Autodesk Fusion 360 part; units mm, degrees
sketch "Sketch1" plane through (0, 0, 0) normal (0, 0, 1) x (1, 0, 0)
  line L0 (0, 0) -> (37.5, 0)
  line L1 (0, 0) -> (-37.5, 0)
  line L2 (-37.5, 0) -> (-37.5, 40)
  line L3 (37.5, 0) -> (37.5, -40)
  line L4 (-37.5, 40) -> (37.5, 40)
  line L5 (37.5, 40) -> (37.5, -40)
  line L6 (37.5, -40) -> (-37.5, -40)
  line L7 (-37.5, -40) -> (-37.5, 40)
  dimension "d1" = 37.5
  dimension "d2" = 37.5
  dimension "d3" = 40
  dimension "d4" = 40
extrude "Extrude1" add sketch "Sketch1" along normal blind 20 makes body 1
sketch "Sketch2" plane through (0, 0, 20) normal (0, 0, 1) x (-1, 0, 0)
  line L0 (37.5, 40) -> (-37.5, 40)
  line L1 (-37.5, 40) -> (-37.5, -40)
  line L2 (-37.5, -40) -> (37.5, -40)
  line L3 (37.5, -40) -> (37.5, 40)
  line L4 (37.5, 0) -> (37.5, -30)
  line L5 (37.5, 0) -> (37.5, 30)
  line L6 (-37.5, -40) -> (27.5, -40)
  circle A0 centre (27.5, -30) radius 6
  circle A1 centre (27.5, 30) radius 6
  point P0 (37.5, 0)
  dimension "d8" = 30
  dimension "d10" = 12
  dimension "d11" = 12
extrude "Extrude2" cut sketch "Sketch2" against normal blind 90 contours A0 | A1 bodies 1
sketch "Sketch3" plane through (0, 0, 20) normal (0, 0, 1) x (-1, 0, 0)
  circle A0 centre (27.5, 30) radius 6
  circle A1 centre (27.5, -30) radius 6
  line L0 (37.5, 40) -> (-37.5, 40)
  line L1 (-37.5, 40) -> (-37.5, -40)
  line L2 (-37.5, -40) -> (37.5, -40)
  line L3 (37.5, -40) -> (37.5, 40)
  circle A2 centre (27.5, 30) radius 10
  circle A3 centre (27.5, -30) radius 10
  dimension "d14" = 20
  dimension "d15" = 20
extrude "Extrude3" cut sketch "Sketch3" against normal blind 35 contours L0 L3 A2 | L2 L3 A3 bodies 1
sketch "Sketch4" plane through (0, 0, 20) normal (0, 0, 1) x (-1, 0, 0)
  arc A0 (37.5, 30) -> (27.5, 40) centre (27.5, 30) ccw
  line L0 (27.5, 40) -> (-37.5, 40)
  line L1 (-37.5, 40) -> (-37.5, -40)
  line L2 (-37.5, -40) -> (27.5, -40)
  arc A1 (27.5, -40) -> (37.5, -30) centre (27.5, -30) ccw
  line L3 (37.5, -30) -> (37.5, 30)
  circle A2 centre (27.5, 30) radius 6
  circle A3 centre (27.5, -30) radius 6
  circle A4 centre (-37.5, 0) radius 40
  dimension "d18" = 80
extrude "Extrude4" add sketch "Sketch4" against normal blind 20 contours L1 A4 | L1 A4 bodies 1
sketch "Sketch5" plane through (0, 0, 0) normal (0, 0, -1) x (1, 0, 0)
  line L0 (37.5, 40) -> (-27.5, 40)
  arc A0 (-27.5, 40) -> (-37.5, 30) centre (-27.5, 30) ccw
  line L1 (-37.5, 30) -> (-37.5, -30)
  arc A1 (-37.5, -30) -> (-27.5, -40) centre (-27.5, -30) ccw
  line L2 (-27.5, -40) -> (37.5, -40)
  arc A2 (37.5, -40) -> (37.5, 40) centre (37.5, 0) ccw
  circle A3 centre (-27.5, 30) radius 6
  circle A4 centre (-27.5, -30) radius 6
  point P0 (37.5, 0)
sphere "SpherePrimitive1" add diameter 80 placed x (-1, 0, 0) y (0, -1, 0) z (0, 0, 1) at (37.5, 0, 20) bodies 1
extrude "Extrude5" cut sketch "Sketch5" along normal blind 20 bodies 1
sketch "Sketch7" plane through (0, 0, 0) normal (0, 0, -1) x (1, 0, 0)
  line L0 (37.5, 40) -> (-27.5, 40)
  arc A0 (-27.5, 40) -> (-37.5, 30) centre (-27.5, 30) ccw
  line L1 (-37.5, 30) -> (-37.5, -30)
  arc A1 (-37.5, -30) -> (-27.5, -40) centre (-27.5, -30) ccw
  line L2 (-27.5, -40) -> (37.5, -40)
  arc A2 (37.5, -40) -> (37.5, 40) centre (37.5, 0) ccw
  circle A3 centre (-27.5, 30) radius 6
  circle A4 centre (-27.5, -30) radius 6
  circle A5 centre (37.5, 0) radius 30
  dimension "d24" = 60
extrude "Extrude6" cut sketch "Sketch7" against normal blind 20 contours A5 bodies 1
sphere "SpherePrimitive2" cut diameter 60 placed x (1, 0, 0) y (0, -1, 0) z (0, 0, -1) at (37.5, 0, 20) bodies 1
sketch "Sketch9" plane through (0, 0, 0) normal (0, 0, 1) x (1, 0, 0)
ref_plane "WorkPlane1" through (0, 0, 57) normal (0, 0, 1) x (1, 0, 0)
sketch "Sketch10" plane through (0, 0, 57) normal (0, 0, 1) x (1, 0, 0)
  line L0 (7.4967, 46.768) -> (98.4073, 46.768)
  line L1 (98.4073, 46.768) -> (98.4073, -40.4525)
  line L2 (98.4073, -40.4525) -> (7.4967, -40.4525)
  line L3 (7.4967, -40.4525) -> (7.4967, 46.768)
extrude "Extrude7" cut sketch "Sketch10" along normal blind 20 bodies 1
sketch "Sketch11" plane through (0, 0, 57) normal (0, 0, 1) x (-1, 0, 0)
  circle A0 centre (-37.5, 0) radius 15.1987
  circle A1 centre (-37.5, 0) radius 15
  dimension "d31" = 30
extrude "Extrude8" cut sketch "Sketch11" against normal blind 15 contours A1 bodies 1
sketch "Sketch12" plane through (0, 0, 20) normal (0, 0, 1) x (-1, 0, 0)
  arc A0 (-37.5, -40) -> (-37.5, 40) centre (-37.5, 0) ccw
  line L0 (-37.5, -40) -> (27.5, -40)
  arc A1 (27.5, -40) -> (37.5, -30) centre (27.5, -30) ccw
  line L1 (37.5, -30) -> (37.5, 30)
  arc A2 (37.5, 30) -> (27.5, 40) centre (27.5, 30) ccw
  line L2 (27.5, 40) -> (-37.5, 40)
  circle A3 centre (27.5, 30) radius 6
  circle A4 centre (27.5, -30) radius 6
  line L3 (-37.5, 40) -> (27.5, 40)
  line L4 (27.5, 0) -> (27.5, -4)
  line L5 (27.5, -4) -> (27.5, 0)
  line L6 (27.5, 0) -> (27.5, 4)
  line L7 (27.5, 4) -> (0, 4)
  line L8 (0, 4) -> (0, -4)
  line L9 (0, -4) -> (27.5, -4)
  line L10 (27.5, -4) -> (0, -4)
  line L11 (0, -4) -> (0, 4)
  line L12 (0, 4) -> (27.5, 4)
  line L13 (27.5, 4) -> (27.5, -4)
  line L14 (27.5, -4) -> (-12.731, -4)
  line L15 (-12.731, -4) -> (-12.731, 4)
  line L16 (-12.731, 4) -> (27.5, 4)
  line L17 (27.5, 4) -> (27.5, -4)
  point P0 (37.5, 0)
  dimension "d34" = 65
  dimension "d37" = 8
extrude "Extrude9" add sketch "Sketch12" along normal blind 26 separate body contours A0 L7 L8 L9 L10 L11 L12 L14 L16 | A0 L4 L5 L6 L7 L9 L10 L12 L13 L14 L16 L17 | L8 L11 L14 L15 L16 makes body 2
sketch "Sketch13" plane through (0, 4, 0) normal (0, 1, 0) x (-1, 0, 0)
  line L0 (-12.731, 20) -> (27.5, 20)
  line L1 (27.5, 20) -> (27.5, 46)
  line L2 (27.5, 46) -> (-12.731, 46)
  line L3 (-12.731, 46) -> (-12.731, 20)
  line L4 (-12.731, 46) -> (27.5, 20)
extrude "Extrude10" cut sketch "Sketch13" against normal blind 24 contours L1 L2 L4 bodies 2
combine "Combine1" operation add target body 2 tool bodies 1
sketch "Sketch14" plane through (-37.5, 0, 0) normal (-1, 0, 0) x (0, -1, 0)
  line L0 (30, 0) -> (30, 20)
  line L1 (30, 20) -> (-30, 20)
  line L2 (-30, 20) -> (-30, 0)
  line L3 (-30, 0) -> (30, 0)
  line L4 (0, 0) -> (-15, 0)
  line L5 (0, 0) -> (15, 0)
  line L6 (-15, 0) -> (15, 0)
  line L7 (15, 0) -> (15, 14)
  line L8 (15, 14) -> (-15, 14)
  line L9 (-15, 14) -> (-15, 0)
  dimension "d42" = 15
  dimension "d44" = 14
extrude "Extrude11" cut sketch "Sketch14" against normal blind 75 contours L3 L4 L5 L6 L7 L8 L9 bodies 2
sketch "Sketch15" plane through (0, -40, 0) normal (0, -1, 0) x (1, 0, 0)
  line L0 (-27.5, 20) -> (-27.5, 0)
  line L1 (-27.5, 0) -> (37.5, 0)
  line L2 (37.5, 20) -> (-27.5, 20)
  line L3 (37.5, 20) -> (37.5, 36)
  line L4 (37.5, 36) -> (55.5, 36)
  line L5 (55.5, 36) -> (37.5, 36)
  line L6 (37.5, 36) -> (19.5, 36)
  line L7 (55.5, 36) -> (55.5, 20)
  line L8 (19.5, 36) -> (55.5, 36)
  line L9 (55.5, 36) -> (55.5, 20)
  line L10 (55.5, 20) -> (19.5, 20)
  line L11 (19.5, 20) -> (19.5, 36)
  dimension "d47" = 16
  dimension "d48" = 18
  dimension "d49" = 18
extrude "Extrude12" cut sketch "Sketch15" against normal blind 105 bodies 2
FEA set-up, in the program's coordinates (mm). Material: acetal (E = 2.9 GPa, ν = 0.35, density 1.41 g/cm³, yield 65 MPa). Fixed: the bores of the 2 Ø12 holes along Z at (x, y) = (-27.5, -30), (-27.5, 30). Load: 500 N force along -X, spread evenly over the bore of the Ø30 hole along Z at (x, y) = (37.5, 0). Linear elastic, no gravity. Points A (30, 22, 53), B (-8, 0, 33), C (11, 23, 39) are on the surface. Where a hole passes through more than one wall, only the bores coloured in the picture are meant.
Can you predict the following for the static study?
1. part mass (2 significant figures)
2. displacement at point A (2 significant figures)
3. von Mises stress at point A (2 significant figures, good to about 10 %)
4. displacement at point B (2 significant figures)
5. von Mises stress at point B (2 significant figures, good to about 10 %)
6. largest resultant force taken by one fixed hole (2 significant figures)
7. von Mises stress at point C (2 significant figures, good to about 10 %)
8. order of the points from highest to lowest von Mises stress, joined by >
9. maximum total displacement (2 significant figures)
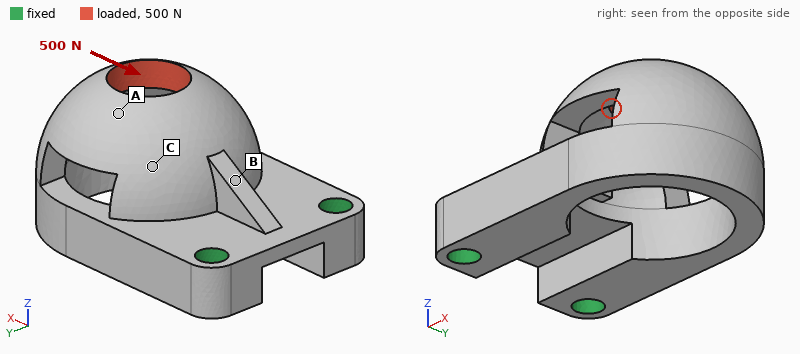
210 g
0.42 mm
0.97 MPa
0.13 mm
6.1 MPa
330 N
1.9 MPa
B > C > A
0.62 mm
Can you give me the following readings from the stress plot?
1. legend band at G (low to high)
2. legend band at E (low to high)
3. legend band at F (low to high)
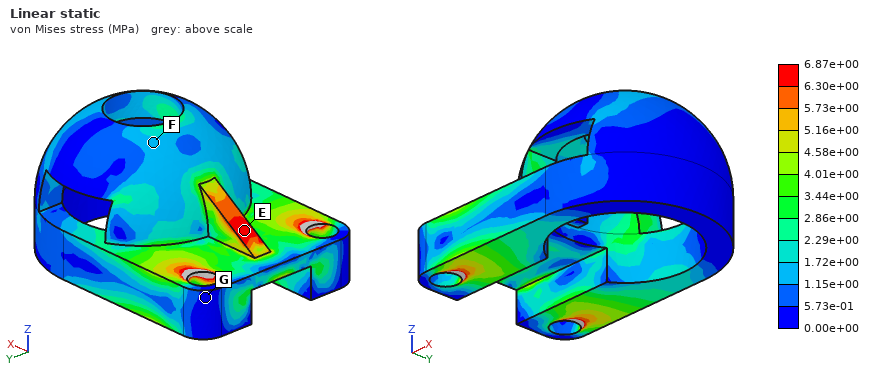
0.00e+00 to 5.73e-01 MPa
6.30e+00 to 6.87e+00 MPa
1.15e+00 to 1.72e+00 MPa
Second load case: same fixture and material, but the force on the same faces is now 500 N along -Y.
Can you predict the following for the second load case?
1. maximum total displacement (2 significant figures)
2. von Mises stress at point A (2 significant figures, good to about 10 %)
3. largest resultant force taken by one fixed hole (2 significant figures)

0.23 mm
1.9 MPa
640 N
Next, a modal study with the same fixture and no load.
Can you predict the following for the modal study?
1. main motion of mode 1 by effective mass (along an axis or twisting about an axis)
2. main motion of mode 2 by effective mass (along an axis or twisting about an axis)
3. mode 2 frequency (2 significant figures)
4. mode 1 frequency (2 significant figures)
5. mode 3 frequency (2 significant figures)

along Z
along Y
710 Hz
390 Hz
1000 Hz
